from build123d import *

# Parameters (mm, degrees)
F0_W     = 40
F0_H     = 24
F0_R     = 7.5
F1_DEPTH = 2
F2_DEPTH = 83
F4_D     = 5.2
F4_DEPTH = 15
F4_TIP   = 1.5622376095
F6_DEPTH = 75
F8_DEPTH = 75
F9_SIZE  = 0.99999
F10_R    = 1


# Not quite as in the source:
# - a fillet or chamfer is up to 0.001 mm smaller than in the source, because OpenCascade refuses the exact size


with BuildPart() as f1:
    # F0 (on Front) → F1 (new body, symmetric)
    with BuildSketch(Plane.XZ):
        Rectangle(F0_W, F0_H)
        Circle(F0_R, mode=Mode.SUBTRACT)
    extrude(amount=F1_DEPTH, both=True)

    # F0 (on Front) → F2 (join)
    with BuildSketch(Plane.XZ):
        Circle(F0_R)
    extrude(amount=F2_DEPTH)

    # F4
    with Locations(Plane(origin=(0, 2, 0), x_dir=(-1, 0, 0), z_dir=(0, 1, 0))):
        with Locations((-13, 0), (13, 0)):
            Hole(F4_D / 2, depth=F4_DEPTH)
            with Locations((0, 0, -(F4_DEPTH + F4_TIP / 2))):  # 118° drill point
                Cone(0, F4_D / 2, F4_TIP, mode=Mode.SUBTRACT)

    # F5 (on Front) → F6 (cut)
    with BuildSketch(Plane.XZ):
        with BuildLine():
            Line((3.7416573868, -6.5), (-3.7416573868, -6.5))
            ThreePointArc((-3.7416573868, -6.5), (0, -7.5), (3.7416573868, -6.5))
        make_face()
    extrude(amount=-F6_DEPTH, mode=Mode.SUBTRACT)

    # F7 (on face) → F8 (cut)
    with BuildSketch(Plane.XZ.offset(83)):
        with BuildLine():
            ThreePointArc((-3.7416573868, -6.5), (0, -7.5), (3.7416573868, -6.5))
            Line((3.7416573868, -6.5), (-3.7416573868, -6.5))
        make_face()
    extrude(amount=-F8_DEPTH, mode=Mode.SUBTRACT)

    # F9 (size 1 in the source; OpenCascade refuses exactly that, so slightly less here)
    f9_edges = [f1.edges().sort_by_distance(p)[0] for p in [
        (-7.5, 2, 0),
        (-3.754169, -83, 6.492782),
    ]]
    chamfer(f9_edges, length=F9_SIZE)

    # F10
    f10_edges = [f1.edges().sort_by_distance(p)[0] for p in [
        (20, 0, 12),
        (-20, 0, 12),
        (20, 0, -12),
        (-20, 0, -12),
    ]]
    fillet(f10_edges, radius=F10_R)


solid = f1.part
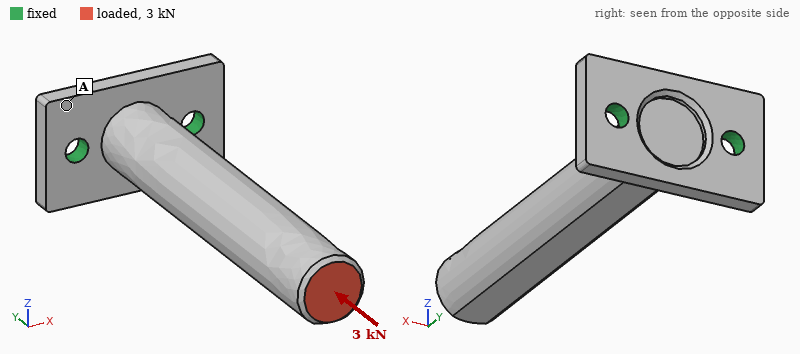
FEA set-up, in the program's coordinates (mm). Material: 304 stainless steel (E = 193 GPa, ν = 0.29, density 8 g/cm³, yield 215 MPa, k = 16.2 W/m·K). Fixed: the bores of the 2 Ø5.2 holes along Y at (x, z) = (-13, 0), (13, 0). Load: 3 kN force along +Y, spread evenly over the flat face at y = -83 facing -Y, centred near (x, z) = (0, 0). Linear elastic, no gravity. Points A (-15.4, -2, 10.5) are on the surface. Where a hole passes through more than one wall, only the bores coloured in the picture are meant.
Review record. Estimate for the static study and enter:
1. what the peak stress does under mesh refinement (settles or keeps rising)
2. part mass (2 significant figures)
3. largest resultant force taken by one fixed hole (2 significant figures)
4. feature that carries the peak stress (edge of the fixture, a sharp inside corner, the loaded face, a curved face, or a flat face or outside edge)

keeps rising
140 g
1.7 kN
edge of the fixture
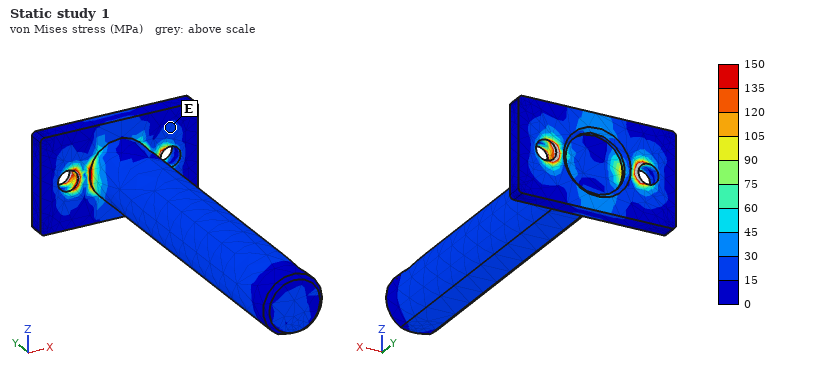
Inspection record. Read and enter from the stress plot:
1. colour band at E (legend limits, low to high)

15 to 30 MPa
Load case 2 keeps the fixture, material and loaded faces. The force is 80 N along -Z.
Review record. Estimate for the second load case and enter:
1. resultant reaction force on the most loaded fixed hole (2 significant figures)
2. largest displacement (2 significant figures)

41 N
94 µm
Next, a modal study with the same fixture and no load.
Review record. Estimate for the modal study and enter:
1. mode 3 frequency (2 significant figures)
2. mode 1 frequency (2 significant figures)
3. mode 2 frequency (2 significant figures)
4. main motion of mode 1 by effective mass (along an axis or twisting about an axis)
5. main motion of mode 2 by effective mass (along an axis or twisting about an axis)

6500 Hz
800 Hz
1200 Hz
along Z
along X
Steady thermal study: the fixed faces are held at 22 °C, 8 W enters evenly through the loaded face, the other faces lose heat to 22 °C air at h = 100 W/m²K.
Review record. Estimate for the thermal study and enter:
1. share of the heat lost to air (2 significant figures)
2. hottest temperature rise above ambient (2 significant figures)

96 %
73 K
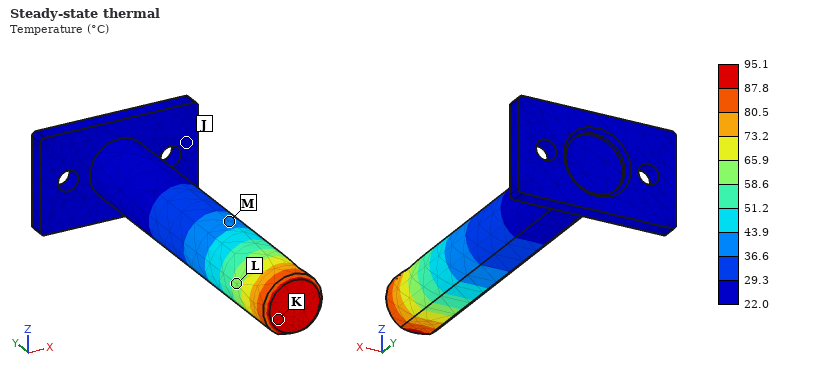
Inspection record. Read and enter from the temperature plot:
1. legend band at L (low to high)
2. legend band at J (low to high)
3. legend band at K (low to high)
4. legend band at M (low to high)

58.6 to 65.9 °C
22.0 to 29.3 °C
87.8 to 95.1 °C
36.6 to 43.9 °C
